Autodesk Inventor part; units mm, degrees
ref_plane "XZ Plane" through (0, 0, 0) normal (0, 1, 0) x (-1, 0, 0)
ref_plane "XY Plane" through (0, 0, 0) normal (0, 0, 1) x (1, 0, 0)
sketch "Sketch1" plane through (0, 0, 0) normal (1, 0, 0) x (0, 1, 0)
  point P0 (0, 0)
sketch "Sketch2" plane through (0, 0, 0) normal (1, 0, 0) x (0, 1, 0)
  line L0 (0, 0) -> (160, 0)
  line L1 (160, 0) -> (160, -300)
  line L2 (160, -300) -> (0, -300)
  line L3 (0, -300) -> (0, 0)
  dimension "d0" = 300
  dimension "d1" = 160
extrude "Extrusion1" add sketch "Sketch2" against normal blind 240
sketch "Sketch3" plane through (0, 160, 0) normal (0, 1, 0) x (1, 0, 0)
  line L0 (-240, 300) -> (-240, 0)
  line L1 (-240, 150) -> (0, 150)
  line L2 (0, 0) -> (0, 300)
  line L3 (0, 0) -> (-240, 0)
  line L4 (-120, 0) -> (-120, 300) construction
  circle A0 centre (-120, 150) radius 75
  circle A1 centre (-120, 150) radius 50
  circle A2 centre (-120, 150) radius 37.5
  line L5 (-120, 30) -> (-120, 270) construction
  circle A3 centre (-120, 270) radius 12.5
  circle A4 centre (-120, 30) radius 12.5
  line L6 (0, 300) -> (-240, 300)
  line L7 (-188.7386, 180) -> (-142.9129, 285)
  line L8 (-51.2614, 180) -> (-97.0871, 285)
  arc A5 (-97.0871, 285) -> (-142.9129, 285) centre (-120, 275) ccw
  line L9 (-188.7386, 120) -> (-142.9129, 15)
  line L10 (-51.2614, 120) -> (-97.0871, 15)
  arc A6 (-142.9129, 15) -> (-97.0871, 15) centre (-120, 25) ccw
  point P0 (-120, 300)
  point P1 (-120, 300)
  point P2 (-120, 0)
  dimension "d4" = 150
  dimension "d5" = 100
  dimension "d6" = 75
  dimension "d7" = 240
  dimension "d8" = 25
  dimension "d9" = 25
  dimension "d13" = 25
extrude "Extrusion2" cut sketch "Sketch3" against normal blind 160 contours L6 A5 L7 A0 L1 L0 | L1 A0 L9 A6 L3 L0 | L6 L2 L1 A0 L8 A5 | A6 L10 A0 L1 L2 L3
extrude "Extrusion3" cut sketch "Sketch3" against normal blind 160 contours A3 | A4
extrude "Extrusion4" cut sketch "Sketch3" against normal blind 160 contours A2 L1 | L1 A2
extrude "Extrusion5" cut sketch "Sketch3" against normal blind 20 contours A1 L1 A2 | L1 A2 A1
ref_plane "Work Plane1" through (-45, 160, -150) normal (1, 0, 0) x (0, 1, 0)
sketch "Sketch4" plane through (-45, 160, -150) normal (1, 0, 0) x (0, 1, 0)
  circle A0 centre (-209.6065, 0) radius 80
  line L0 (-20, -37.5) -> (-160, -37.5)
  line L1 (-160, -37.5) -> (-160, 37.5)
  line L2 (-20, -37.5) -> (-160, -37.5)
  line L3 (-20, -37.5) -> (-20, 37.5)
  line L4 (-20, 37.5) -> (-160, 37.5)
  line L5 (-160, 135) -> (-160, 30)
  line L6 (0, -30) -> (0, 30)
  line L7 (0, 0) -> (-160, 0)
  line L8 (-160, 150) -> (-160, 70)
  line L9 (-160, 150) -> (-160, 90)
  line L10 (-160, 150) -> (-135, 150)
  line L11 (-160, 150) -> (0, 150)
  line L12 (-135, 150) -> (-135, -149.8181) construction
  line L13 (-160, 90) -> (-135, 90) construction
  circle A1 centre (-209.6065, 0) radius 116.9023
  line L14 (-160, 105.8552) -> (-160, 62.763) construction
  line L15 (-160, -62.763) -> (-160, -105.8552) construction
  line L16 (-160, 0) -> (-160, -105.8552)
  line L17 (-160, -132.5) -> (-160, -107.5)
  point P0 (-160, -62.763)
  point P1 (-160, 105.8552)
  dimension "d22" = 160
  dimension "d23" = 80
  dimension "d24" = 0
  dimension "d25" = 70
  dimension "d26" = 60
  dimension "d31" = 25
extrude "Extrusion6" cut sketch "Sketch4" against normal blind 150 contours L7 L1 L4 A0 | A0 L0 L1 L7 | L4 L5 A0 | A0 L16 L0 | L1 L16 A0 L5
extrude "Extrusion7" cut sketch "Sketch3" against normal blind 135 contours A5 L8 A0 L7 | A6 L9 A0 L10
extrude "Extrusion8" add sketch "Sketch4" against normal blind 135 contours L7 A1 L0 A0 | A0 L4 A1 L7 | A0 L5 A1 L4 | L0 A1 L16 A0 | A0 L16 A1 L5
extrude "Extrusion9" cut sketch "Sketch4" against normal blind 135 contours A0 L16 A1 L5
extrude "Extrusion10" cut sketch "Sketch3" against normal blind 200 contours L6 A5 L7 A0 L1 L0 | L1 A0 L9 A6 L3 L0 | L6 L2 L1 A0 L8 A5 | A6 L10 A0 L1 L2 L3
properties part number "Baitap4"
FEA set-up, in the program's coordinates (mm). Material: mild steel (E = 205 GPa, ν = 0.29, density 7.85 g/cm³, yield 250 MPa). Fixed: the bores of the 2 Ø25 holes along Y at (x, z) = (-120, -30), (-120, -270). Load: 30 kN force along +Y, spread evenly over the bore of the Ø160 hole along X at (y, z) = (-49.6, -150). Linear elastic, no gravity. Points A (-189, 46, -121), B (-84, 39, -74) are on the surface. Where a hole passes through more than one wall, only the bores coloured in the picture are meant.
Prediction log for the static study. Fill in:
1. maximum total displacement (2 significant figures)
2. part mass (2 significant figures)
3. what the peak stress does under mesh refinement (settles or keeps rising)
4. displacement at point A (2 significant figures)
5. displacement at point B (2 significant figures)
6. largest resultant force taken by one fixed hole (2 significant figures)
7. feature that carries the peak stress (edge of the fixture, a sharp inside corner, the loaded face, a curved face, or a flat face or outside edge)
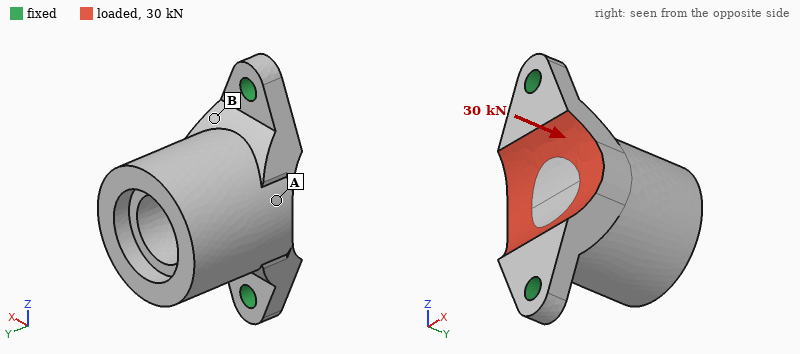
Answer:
14 µm
18 kg
keeps rising
13 µm
10 µm
20 kN
edge of the fixture
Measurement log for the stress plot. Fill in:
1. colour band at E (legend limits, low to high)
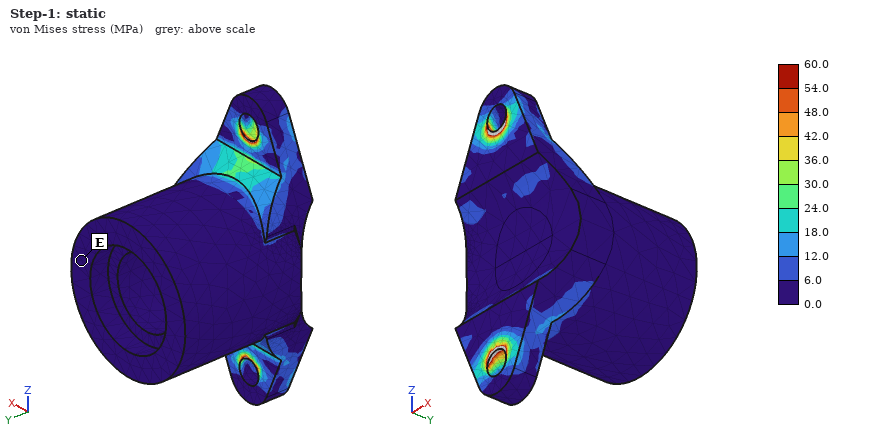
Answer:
0.0 to 6.0 MPa
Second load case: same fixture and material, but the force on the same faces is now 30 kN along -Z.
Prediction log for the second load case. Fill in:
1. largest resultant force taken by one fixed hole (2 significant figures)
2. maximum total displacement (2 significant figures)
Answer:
15 kN
4.1 µm
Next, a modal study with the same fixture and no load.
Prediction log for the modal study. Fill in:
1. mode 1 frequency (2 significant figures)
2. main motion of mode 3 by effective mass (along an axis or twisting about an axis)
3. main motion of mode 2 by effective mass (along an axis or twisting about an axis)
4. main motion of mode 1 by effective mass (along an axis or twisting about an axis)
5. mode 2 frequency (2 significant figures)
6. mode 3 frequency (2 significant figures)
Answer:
540 Hz
along Z
along Y
along X
1900 Hz
2000 Hz
